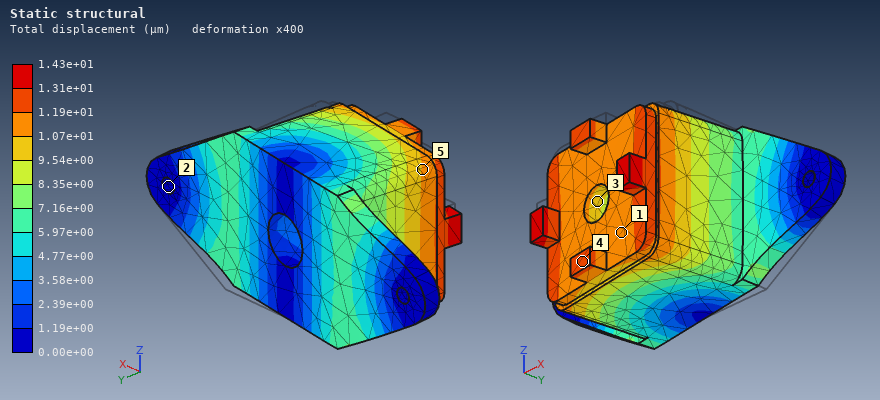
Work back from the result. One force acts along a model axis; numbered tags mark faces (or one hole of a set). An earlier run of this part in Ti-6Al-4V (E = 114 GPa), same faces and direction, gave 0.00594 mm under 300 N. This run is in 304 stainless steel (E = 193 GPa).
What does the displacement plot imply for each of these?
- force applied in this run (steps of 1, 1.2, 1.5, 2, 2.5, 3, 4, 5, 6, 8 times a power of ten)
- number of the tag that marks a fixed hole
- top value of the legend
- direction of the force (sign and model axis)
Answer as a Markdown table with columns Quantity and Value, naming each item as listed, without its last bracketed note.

| Quantity | Value |
|---|---|
| force applied in this run | 1.2 kN |
| number of the tag that marks a fixed hole | 2 |
| top value of the legend | 1.43e+01 µm |
| direction of the force | -X |
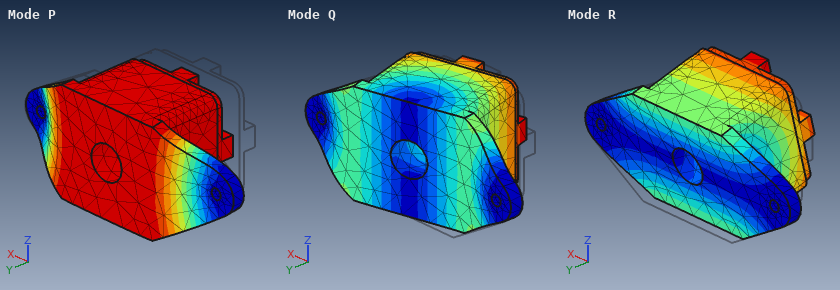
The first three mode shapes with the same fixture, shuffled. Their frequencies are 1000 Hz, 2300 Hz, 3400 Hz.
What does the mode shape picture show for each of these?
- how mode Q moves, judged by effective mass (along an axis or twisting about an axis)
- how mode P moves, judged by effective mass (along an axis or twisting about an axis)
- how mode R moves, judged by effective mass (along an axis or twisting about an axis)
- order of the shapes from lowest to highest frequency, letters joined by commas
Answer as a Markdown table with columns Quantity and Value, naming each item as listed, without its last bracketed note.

| Quantity | Value |
|---|---|
| how mode Q moves, judged by effective mass | along X |
| how mode P moves, judged by effective mass | along Y |
| how mode R moves, judged by effective mass | along Z |
| order of the shapes from lowest to highest frequency, letters joined by commas | R, P, Q |
